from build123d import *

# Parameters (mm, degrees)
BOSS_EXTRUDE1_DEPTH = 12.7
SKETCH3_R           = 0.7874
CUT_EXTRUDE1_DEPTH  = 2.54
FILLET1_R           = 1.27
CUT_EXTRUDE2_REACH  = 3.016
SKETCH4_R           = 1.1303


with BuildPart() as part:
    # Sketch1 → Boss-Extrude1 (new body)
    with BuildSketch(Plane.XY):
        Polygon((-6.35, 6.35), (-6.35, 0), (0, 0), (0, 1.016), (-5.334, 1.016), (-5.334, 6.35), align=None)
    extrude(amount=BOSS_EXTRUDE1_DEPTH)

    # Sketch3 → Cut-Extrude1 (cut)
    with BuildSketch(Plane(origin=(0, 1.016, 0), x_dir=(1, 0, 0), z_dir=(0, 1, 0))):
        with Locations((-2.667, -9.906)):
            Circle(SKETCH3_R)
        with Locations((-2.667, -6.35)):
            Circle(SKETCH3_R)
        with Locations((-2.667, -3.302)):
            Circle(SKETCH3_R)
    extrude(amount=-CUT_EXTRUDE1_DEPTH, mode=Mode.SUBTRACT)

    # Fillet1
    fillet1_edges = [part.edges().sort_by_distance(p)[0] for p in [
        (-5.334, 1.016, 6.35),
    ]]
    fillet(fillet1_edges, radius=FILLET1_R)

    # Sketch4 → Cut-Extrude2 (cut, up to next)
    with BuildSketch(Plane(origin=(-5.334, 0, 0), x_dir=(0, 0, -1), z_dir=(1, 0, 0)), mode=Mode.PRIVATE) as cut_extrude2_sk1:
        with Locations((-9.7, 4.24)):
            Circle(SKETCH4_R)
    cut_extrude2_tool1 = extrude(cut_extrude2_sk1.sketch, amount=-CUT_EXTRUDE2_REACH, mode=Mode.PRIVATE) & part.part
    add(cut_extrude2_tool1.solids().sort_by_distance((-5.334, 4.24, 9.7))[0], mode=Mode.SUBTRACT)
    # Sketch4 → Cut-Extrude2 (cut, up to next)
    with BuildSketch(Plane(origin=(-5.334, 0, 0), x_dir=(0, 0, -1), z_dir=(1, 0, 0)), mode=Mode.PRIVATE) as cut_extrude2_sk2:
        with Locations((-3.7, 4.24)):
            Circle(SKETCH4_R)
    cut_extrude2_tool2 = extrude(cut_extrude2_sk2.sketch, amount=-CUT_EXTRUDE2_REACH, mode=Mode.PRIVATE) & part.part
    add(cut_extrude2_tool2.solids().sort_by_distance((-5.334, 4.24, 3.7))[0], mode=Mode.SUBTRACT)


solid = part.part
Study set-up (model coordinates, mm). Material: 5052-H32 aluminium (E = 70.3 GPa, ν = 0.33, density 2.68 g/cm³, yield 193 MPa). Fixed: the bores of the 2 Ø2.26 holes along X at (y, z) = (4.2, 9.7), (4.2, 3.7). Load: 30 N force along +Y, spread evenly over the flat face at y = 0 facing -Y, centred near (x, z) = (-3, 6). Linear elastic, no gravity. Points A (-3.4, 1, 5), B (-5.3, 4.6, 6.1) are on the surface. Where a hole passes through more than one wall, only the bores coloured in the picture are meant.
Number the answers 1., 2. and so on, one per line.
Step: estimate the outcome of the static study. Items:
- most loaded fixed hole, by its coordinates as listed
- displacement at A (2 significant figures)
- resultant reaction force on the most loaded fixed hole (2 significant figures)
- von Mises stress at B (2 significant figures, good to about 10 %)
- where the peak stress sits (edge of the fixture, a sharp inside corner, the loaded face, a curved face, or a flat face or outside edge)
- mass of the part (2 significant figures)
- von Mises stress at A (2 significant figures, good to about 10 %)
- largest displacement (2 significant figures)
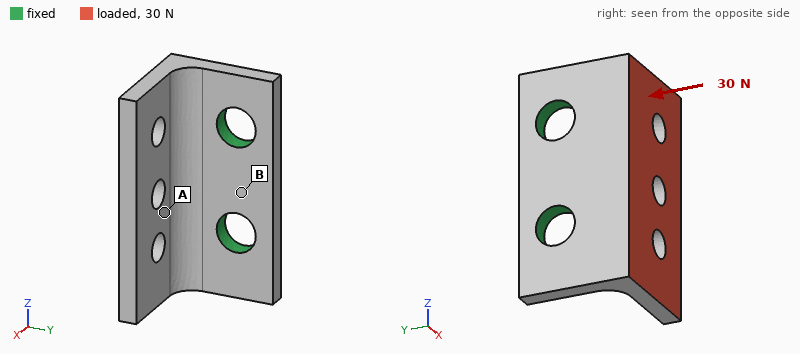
1. (4.2, 3.7)
2. 6.5 µm
3. 16 N
4. 6.5 MPa
5. a flat face or outside edge
6. 0.38 g
7. 18 MPa
8. 19 µm
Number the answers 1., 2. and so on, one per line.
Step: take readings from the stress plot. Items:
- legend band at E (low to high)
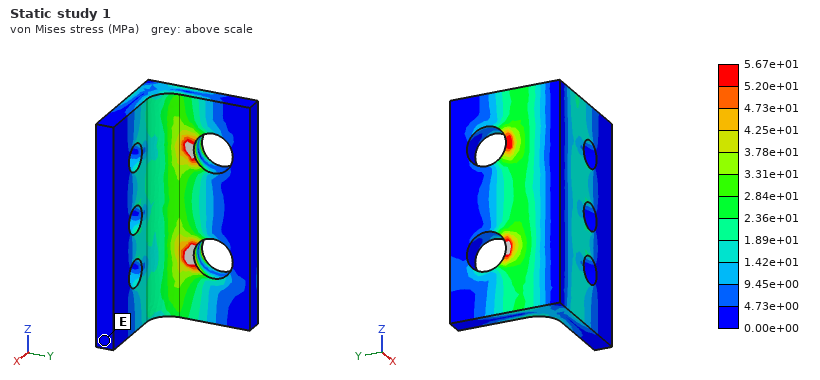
1. 0.00e+00 to 4.73e+00 MPa
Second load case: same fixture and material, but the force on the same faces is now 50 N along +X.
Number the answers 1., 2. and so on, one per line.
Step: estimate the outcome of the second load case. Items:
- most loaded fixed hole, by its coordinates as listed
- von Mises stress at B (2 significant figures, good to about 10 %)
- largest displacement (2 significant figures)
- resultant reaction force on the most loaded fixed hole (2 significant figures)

1. (4.2, 3.7)
2. 13 MPa
3. 24 µm
4. 27 N
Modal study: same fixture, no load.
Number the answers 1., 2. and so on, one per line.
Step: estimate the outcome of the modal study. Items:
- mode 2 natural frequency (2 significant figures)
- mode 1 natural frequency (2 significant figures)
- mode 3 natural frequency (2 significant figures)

1. 24 kHz
2. 16 kHz
3. 42 kHz
